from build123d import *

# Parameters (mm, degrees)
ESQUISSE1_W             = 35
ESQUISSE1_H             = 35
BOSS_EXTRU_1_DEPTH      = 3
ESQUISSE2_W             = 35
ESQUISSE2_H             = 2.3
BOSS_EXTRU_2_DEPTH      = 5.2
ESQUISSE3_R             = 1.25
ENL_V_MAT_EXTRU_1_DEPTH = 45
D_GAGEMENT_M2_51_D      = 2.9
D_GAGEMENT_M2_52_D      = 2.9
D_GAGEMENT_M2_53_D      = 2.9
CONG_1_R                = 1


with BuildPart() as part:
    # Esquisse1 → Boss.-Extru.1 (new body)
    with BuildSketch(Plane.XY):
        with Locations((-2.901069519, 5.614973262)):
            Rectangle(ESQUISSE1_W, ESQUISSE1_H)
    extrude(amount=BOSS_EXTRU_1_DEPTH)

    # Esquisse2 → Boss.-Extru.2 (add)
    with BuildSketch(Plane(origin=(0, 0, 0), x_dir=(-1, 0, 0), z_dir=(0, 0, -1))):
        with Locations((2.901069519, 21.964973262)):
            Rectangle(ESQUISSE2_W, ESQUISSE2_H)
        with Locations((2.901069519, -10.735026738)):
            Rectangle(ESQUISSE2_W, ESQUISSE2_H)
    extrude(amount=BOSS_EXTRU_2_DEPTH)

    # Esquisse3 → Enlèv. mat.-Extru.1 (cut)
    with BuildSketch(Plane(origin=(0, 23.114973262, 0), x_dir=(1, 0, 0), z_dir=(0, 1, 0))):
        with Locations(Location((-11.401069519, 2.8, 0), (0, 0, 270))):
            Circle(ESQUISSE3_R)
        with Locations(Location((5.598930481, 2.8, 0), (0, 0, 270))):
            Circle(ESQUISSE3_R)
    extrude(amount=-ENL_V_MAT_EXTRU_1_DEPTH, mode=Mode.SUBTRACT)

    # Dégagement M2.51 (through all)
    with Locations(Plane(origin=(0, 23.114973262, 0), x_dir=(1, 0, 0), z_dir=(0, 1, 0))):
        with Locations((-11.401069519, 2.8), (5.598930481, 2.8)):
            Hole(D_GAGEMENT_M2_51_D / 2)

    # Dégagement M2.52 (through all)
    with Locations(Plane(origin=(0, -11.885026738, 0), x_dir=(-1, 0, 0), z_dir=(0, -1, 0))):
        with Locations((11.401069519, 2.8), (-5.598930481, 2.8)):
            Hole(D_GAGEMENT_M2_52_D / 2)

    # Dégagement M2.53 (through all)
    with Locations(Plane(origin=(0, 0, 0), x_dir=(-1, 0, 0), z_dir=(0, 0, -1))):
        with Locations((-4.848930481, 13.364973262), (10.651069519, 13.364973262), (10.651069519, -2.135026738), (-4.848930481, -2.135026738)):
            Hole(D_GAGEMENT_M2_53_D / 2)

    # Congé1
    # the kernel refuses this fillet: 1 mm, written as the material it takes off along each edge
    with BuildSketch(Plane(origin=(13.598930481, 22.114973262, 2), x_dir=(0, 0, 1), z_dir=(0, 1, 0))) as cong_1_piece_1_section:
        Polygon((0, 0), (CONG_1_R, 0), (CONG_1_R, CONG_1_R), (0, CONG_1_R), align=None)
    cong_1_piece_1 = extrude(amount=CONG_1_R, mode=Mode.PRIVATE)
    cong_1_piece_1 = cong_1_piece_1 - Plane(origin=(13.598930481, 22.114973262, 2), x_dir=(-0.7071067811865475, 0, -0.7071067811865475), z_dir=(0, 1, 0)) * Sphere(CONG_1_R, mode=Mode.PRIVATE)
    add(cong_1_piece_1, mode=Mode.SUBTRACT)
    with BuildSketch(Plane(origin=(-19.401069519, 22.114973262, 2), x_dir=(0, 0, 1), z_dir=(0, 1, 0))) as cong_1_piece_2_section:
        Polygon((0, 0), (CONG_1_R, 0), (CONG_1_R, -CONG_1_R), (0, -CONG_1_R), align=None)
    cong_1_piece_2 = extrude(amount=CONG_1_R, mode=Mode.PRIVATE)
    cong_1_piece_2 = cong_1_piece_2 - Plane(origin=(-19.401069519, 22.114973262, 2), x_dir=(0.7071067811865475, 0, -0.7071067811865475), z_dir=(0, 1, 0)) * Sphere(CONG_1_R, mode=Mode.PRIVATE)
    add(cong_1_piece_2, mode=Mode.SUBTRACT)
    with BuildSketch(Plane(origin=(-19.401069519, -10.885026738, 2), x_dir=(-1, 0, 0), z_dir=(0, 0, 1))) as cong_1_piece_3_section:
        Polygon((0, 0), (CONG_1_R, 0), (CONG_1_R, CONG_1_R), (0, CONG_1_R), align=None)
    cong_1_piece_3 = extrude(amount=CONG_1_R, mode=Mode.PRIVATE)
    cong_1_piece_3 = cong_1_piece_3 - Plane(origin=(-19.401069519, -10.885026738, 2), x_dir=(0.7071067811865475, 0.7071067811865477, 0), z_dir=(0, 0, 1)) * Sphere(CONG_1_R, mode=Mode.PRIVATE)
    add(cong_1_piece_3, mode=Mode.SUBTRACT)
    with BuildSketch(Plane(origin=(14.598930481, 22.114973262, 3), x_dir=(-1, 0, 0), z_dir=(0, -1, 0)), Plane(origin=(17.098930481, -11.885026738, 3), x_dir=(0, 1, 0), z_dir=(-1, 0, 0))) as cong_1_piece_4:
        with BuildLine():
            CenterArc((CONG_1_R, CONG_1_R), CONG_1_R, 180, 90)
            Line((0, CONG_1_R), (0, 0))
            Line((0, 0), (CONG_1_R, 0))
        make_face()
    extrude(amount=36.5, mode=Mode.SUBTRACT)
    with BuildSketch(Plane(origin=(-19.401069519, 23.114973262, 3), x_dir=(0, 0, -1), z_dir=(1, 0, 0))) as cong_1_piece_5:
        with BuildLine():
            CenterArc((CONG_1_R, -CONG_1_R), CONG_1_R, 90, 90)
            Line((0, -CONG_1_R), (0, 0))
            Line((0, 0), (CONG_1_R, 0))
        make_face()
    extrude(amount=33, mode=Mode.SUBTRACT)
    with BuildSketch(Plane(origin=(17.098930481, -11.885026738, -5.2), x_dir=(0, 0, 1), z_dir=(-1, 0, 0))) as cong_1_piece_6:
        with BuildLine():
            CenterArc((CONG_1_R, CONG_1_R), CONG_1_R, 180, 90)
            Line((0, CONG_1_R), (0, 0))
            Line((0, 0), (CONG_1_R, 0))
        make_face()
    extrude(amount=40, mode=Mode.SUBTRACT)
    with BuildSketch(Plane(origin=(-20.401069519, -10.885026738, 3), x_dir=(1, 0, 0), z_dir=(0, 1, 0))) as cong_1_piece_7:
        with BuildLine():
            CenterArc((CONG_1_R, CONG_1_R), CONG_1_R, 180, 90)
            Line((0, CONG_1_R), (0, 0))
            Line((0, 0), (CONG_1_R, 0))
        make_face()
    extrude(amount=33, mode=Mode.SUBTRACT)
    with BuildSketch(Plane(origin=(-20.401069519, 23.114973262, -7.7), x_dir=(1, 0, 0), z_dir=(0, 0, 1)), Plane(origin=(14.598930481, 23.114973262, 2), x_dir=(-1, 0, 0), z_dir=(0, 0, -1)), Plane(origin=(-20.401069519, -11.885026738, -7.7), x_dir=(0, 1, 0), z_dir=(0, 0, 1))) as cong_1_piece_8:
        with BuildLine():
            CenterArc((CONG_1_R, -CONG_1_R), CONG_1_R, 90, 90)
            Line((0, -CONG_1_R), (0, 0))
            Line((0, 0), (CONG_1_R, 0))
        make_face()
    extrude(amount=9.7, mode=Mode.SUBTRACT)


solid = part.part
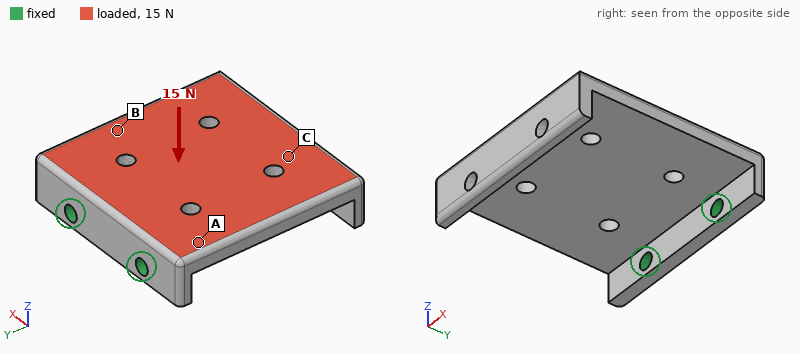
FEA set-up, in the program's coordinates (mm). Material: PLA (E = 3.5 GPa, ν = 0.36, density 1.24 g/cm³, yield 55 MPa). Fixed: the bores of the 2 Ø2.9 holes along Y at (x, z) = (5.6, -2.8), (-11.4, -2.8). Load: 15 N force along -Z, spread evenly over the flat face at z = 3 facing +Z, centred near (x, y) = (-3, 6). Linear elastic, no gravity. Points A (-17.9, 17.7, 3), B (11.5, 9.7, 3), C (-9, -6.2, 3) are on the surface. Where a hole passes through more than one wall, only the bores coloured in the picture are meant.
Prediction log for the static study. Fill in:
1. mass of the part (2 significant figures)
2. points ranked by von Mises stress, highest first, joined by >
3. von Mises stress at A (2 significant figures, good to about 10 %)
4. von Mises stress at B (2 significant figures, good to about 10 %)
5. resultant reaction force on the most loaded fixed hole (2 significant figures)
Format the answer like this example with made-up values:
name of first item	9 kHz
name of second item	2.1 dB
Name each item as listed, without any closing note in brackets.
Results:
mass of the part	5.4 g
points ranked by von Mises stress, highest first, joined by >	A > B > C
von Mises stress at A	3.4 MPa
von Mises stress at B	2.0 MPa
resultant reaction force on the most loaded fixed hole	7.8 N
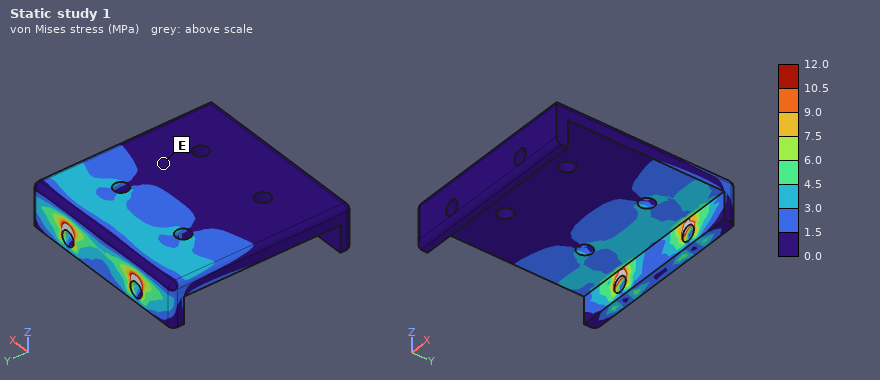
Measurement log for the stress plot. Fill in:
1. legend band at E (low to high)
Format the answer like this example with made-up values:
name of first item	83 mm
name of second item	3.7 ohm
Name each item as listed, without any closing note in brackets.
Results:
legend band at E	0.0 to 1.5 MPa
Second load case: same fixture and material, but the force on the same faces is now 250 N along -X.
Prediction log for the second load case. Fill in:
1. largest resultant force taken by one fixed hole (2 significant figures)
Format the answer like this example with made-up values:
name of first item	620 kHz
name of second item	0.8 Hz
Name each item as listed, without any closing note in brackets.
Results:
largest resultant force taken by one fixed hole	260 N
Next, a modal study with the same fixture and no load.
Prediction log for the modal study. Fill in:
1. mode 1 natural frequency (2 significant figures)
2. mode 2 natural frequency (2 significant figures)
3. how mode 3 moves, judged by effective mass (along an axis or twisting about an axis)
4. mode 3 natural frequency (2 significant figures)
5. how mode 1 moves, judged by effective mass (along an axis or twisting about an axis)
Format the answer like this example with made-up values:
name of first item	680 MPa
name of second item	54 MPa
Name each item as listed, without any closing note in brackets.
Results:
mode 1 natural frequency	430 Hz
mode 2 natural frequency	1200 Hz
how mode 3 moves, judged by effective mass	along X
mode 3 natural frequency	2000 Hz
how mode 1 moves, judged by effective mass	along Z
